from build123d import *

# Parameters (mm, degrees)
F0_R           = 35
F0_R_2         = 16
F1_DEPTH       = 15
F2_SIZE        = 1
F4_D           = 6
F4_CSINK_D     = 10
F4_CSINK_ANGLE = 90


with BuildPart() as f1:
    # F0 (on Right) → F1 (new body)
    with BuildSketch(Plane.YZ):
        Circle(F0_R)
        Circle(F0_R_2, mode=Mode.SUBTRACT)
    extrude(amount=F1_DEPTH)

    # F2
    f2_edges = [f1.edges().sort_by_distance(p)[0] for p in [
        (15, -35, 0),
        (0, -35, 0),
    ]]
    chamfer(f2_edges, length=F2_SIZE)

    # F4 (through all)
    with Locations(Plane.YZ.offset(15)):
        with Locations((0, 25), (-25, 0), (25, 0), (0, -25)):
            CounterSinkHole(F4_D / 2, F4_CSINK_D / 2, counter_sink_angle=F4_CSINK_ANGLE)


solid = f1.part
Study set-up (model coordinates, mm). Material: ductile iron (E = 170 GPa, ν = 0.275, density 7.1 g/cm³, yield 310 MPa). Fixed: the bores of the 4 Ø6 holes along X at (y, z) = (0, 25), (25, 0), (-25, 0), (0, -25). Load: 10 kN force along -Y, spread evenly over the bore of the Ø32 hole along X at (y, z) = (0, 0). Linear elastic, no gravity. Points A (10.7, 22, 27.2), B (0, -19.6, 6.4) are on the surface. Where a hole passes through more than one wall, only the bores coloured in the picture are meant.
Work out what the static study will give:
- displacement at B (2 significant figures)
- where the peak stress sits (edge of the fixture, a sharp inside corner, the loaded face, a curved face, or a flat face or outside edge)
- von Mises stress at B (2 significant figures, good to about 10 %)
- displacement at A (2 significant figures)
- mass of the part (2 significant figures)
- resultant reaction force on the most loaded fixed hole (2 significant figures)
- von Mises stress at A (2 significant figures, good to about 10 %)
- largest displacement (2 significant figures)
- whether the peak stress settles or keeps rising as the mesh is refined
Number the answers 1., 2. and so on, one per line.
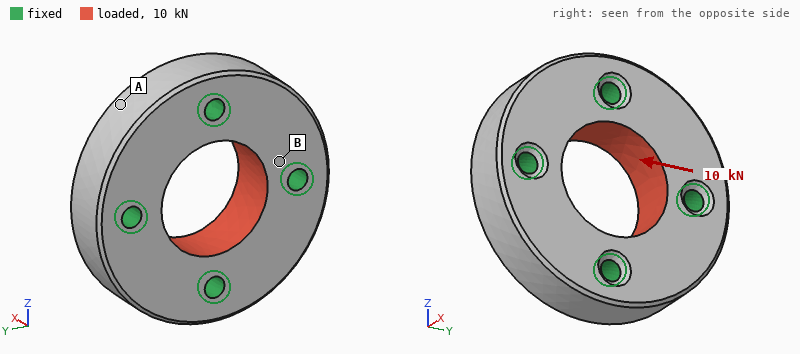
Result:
1. 0.51 µm
2. edge of the fixture
3. 8.7 MPa
4. 0.59 µm
5. 310 g
6. 2.5 kN
7. 4.2 MPa
8. 1.1 µm
9. keeps rising
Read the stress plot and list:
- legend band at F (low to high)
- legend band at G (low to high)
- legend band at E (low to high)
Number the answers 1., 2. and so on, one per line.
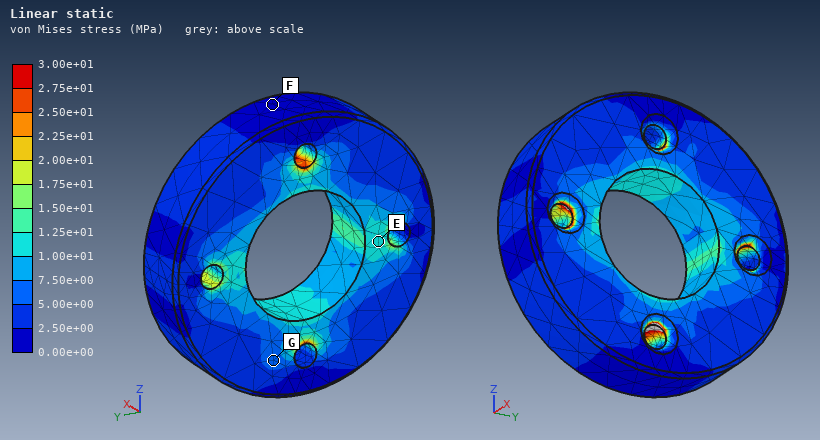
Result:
1. 0.00e+00 to 2.50e+00 MPa
2. 5.00e+00 to 7.50e+00 MPa
3. 1.00e+01 to 1.25e+01 MPa
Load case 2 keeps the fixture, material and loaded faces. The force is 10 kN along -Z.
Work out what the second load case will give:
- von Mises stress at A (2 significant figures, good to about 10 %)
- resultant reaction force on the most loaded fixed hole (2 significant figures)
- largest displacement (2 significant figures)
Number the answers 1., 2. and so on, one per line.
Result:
1. 4.4 MPa
2. 2.5 kN
3. 1.1 µm
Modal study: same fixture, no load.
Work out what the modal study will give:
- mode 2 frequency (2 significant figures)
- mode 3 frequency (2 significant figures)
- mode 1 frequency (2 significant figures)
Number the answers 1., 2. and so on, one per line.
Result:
1. 23 kHz
2. 23 kHz
3. 22 kHz
